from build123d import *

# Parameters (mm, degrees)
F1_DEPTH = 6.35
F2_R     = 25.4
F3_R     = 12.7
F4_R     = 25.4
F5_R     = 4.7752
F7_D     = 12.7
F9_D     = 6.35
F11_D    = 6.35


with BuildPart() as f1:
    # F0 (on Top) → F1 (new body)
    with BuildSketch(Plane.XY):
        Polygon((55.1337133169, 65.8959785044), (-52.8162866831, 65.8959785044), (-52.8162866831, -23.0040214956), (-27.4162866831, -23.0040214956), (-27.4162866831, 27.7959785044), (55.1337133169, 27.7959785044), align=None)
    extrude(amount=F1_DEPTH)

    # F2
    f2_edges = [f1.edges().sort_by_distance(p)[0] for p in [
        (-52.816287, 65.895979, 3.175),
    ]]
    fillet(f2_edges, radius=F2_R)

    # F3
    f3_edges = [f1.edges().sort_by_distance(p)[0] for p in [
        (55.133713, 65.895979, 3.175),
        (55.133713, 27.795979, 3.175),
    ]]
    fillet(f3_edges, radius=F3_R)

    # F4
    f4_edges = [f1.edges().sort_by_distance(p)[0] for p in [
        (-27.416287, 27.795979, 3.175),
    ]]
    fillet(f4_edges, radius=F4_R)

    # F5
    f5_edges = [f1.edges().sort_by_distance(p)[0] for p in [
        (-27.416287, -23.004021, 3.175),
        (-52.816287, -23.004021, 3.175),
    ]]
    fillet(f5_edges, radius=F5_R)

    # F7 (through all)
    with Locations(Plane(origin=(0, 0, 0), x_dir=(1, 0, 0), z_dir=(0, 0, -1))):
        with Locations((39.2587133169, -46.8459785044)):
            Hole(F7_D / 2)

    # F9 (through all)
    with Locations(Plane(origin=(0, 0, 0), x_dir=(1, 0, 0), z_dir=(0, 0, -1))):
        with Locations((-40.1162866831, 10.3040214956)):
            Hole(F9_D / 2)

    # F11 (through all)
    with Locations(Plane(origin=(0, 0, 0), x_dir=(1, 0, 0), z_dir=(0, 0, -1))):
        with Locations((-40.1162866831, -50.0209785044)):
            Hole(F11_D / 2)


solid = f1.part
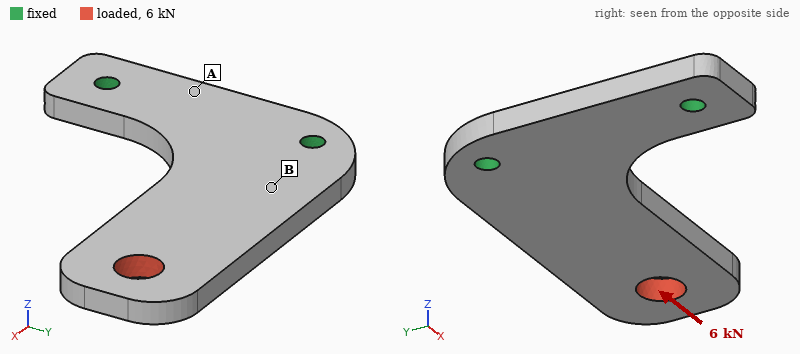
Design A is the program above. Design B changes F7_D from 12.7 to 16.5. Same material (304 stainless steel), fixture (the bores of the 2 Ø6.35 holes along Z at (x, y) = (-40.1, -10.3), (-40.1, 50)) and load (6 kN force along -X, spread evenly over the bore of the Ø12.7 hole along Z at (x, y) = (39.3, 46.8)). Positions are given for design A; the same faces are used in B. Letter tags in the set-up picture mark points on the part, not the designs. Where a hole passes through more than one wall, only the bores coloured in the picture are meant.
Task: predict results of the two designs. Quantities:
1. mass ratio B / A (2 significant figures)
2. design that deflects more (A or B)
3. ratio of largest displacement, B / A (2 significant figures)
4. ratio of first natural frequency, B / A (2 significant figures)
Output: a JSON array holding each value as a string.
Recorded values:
["0.98", "B", "1.1", "1.0"]
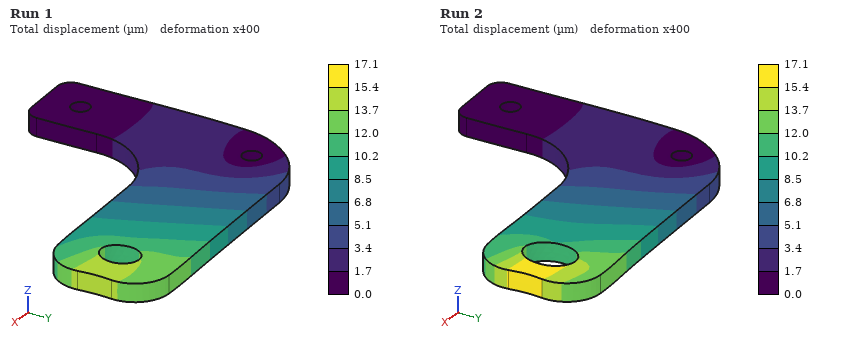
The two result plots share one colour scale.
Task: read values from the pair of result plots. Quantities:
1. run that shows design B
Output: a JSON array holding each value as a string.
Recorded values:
["Run 2"]
